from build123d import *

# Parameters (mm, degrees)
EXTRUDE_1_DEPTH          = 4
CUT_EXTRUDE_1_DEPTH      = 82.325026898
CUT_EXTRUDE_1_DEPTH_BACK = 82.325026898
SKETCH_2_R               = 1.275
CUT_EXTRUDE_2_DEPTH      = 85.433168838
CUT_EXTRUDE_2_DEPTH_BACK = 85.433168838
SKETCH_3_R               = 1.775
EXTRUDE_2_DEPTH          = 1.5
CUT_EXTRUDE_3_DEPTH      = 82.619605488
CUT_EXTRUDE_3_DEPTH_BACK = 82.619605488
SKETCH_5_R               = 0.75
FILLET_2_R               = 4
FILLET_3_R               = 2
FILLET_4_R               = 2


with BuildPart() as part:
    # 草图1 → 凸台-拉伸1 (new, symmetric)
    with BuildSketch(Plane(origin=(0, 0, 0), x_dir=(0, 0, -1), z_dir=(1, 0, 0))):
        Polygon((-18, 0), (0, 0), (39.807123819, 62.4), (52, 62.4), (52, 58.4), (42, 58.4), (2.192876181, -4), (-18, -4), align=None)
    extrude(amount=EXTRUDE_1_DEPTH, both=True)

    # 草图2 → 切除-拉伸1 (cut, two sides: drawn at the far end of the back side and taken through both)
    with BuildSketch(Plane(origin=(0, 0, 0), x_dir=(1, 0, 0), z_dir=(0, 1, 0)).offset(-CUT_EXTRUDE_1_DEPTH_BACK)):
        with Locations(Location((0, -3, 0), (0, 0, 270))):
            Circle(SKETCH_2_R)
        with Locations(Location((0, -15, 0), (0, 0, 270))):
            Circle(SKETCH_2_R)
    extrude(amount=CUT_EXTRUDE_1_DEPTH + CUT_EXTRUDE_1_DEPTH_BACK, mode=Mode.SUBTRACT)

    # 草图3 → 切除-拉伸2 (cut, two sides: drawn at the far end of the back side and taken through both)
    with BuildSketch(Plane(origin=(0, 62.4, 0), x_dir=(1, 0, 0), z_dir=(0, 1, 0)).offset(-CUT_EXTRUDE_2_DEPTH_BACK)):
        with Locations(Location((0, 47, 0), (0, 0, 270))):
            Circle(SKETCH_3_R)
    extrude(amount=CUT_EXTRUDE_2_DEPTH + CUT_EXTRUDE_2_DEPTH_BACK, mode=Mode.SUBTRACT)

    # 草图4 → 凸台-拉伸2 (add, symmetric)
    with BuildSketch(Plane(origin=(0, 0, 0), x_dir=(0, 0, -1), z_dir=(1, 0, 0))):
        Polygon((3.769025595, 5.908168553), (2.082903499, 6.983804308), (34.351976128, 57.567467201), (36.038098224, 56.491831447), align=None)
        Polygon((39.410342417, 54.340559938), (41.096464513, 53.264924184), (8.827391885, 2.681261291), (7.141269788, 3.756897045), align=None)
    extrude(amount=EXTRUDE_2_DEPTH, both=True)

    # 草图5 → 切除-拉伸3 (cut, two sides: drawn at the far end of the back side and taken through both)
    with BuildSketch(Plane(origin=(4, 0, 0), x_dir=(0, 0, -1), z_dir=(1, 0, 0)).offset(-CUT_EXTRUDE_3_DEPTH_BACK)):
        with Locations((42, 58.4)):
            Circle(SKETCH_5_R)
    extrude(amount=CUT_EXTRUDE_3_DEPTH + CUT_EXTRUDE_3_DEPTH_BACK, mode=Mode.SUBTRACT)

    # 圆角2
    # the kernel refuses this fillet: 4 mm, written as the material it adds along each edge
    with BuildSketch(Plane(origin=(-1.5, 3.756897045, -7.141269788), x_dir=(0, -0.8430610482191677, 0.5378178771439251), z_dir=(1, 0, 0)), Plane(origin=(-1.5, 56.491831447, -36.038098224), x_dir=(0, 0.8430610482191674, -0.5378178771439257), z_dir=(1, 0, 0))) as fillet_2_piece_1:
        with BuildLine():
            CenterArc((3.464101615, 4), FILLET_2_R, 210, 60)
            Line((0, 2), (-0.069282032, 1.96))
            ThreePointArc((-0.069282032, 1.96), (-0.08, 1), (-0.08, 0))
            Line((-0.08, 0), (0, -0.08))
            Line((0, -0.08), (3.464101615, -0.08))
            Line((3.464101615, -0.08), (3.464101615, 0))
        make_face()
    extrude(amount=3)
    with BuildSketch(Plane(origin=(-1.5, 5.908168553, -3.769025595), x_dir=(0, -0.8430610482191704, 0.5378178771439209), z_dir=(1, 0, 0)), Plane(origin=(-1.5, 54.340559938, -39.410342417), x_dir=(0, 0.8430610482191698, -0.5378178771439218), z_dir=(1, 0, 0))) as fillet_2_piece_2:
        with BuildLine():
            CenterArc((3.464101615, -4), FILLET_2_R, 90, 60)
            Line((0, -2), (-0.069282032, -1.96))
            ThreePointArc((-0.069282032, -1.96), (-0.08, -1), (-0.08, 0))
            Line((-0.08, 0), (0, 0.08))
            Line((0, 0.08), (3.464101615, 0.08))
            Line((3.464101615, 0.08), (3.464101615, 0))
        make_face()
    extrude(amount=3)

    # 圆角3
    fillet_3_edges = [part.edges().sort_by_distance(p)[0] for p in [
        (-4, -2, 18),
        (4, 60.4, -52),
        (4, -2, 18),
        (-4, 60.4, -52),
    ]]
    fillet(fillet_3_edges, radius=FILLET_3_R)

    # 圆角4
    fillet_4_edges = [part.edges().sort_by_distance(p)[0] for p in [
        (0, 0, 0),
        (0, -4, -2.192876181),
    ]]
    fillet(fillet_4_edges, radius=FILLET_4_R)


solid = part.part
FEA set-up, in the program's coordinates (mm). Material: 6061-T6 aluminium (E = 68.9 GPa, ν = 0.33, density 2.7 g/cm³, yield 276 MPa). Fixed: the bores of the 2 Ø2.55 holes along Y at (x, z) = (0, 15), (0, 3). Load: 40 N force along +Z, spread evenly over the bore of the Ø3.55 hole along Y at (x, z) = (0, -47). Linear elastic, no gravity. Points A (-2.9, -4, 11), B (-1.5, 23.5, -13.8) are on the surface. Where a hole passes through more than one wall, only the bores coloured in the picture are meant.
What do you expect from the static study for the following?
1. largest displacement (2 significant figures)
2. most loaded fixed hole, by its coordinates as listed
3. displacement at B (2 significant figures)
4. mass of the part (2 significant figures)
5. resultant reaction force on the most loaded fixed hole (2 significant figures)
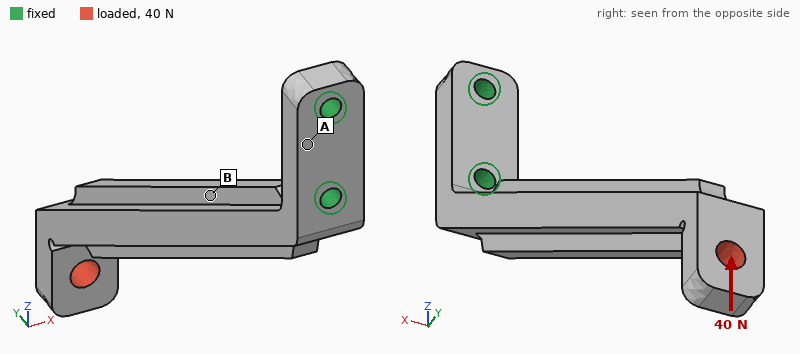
1.1 mm
(0, 3)
0.27 mm
11 g
51 N
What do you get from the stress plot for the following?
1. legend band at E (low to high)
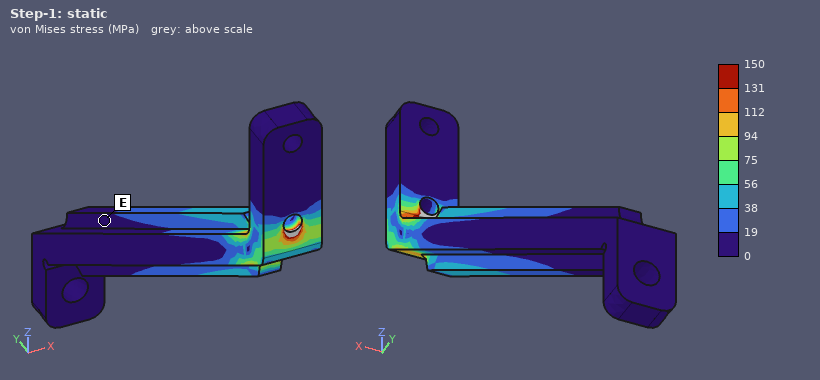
0 to 19 MPa
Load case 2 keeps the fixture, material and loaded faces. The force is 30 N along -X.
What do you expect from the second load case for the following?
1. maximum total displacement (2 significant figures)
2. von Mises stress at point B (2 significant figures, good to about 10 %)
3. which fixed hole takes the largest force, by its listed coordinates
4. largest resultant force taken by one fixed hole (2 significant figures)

0.57 mm
12 MPa
(0, 3)
92 N
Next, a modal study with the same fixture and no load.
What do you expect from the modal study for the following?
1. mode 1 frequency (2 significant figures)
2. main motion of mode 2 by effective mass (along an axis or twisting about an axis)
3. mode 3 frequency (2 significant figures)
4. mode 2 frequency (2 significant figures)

530 Hz
along X
4000 Hz
730 Hz
